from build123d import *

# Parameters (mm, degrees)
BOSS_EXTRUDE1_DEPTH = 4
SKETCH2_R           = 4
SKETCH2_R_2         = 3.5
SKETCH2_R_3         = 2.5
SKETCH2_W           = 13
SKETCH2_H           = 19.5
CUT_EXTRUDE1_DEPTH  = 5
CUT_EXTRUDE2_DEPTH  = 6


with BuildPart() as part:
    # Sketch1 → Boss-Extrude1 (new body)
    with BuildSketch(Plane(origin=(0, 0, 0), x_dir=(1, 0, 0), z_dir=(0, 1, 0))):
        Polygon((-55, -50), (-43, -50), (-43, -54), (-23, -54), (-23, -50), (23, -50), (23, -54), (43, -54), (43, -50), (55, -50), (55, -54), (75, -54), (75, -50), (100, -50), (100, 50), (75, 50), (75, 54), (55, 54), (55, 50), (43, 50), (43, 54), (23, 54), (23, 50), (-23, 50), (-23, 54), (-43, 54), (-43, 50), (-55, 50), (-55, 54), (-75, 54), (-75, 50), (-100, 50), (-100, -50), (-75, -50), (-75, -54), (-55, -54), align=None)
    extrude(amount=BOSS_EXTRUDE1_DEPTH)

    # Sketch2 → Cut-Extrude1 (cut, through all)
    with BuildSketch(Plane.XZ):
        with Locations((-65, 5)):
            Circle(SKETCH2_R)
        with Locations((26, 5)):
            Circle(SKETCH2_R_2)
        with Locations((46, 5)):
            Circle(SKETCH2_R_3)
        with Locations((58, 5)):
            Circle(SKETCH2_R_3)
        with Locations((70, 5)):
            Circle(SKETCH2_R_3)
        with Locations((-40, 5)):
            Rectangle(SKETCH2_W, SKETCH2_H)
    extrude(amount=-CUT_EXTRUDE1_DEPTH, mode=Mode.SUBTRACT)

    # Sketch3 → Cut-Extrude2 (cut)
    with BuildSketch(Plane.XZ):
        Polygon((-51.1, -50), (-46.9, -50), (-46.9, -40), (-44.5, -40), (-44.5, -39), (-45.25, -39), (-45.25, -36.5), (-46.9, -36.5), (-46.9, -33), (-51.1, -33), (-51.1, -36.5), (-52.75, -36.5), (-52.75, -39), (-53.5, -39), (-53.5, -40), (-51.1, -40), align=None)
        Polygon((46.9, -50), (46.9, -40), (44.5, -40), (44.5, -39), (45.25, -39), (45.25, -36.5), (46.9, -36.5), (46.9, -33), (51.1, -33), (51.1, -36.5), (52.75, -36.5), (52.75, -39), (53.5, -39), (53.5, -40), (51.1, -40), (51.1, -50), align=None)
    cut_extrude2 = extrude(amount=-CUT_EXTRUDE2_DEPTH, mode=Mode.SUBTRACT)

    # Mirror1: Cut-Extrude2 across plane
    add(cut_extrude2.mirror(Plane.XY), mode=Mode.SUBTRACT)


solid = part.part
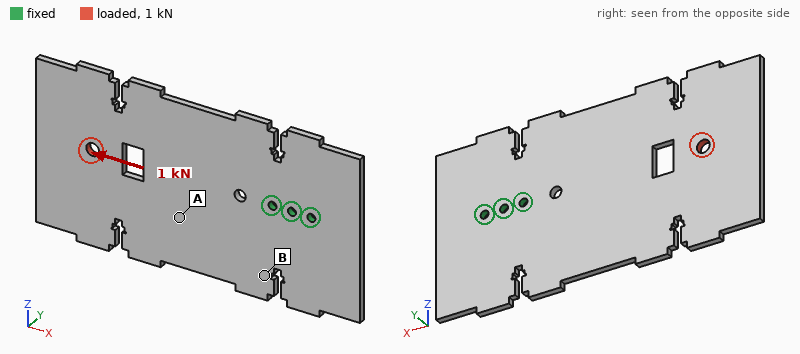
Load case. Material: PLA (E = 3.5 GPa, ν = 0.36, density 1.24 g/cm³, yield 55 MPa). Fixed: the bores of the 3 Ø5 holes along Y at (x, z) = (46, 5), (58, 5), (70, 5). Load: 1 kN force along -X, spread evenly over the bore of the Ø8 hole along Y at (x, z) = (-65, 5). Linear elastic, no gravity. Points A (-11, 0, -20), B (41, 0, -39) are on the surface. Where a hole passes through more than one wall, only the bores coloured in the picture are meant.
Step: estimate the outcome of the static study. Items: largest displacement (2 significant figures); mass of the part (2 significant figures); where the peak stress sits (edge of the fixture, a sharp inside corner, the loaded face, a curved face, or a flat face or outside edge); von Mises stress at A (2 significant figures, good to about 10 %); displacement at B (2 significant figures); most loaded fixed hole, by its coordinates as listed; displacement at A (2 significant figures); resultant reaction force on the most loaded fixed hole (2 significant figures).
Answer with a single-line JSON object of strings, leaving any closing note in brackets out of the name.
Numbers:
{"largest displacement": "0.20 mm", "mass of the part": "99 g", "where the peak stress sits": "the loaded face", "von Mises stress at A": "3.2 MPa", "displacement at B": "0.050 mm", "most loaded fixed hole, by its coordinates as listed": "(46, 5)", "displacement at A": "0.074 mm", "resultant reaction force on the most loaded fixed hole": "510 N"}
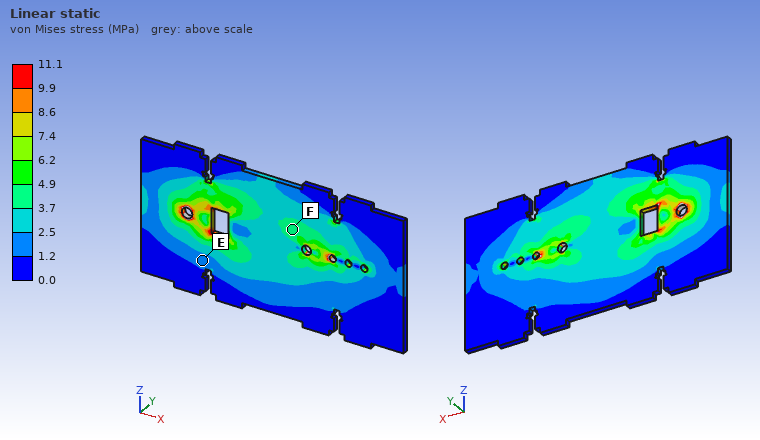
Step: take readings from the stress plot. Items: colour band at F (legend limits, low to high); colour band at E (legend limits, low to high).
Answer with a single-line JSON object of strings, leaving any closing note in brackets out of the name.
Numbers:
{"colour band at F": "3.7 to 4.9 MPa", "colour band at E": "1.2 to 2.5 MPa"}
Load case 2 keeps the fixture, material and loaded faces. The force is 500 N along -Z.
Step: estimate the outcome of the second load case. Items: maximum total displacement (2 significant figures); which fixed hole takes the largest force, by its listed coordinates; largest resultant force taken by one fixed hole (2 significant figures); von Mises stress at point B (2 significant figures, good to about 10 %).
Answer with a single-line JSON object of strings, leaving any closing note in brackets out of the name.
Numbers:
{"maximum total displacement": "2.6 mm", "which fixed hole takes the largest force, by its listed coordinates": "(46, 5)", "largest resultant force taken by one fixed hole": "2.4 kN", "von Mises stress at point B": "6.2 MPa"}
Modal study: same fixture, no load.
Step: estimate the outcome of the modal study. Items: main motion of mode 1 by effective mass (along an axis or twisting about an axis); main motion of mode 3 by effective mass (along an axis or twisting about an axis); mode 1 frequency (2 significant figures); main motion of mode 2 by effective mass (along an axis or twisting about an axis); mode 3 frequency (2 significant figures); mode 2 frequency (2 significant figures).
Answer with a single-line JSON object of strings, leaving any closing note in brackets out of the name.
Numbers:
{"main motion of mode 1 by effective mass": "along Y", "main motion of mode 3 by effective mass": "along Y", "mode 1 frequency": "46 Hz", "main motion of mode 2 by effective mass": "twisting about X", "mode 3 frequency": "250 Hz", "mode 2 frequency": "120 Hz"}
